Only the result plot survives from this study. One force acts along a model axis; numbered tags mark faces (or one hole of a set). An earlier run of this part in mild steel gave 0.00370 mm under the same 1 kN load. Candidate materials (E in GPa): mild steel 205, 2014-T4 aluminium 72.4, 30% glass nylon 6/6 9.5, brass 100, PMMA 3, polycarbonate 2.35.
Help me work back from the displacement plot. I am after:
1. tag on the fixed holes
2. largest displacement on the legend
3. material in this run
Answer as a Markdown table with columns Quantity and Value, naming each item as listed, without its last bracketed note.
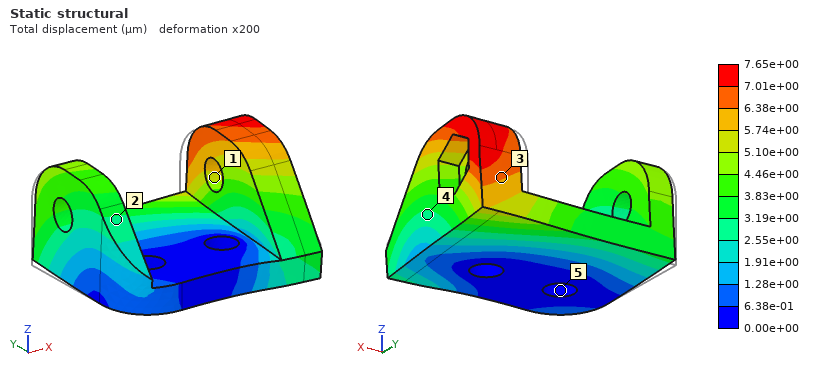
| Quantity | Value |
|---|---|
| tag on the fixed holes | 5 |
| largest displacement on the legend | 7.65e+00 µm |
| material in this run | brass |
